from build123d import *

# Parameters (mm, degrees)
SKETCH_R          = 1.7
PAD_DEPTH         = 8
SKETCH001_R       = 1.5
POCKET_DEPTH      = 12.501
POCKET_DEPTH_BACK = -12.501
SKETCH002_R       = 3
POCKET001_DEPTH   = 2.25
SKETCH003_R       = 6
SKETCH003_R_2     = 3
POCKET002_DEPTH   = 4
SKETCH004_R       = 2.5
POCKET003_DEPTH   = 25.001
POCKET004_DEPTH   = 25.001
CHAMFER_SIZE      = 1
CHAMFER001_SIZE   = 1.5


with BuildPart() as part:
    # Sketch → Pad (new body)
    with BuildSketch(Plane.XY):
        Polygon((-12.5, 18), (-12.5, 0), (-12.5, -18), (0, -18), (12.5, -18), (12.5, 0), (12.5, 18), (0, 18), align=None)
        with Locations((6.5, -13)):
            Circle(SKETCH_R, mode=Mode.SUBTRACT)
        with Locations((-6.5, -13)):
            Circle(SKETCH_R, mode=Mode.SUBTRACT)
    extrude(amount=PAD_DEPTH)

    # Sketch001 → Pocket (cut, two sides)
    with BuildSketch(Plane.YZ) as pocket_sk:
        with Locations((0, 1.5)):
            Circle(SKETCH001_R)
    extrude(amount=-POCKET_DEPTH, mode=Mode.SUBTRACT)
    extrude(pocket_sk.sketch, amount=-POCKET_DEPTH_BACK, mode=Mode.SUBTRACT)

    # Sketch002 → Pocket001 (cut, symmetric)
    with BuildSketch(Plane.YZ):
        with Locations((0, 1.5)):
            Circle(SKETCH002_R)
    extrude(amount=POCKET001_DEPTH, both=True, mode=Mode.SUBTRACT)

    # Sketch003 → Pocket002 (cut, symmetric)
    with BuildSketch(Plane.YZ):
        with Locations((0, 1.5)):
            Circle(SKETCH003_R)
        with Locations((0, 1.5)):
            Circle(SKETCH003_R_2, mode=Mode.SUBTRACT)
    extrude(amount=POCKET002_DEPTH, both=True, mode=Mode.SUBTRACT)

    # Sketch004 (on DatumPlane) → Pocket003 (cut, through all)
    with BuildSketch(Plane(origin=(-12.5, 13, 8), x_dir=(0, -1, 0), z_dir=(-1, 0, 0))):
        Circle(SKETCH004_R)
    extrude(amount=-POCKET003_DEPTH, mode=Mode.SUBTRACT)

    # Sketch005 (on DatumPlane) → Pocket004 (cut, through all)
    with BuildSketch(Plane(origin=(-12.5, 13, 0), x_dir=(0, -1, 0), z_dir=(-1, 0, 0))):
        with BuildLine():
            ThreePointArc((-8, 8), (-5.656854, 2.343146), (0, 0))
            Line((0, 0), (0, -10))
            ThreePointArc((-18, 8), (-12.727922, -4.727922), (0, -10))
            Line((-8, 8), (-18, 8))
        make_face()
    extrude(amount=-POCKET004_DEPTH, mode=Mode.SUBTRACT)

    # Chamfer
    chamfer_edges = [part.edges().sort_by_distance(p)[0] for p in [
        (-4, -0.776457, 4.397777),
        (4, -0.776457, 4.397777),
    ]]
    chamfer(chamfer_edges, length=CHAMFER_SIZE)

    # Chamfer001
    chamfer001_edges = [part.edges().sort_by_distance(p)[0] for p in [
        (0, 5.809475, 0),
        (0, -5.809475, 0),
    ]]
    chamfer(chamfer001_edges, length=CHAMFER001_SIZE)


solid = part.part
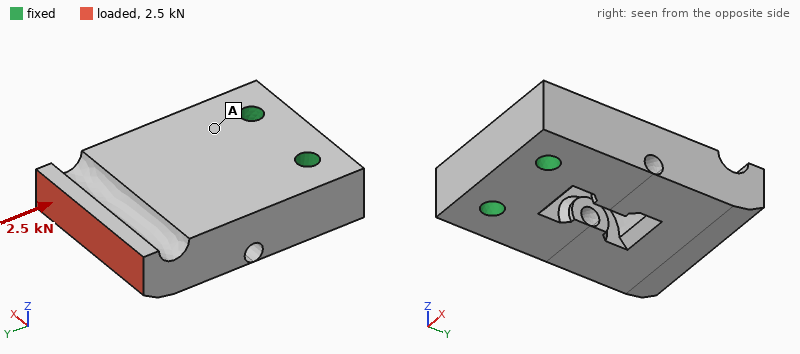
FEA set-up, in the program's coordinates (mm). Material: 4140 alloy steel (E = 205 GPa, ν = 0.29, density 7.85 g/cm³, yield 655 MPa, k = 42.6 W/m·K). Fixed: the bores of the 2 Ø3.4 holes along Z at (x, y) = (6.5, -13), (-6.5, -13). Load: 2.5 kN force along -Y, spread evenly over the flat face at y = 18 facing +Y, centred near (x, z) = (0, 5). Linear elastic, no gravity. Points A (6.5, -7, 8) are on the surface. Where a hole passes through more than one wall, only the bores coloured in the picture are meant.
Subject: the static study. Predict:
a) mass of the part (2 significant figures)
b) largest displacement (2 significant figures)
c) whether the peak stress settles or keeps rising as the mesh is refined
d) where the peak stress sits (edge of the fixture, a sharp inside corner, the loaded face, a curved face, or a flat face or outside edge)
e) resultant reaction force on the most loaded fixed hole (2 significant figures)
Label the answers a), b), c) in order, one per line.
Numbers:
a) 48 g
b) 6.4 µm
c) keeps rising
d) a sharp inside corner
e) 1.3 kN
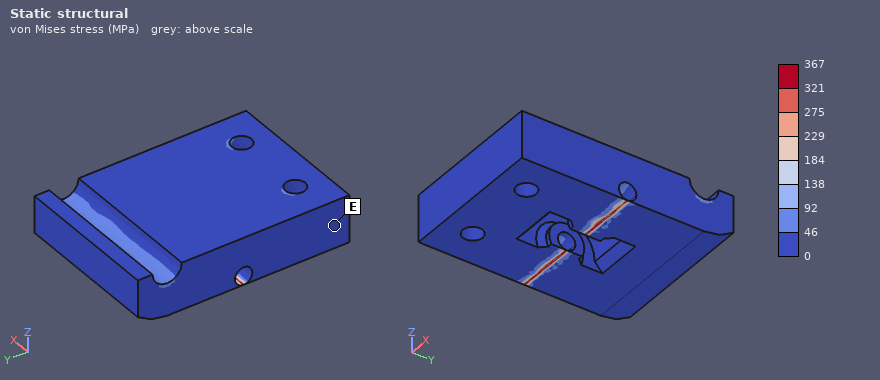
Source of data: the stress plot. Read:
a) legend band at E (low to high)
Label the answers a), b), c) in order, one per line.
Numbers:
a) 0 to 46 MPa
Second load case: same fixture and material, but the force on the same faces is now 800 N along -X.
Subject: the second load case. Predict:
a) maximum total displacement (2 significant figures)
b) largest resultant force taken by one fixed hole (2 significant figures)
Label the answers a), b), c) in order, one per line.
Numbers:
a) 11 µm
b) 1.6 kN
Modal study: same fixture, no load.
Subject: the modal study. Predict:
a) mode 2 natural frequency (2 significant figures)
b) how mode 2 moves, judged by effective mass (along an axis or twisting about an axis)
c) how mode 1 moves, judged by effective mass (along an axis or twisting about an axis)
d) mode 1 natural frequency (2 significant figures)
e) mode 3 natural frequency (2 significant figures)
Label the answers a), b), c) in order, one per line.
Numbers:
a) 12 kHz
b) along X
c) along Z
d) 5700 Hz
e) 14 kHz
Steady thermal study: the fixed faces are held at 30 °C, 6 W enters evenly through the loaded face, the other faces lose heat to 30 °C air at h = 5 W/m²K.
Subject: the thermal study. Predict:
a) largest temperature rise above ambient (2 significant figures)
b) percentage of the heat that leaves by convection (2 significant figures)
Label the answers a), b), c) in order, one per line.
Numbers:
a) 31 K
b) 3.0 %
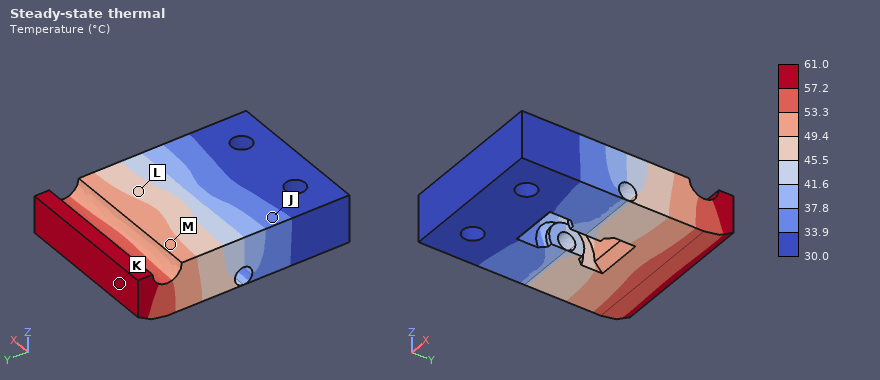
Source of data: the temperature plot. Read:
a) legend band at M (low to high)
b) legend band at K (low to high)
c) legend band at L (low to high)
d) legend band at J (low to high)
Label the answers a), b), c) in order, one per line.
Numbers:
a) 49.4 to 53.3 °C
b) 57.2 to 61.0 °C
c) 45.5 to 49.4 °C
d) 33.9 to 37.8 °C
